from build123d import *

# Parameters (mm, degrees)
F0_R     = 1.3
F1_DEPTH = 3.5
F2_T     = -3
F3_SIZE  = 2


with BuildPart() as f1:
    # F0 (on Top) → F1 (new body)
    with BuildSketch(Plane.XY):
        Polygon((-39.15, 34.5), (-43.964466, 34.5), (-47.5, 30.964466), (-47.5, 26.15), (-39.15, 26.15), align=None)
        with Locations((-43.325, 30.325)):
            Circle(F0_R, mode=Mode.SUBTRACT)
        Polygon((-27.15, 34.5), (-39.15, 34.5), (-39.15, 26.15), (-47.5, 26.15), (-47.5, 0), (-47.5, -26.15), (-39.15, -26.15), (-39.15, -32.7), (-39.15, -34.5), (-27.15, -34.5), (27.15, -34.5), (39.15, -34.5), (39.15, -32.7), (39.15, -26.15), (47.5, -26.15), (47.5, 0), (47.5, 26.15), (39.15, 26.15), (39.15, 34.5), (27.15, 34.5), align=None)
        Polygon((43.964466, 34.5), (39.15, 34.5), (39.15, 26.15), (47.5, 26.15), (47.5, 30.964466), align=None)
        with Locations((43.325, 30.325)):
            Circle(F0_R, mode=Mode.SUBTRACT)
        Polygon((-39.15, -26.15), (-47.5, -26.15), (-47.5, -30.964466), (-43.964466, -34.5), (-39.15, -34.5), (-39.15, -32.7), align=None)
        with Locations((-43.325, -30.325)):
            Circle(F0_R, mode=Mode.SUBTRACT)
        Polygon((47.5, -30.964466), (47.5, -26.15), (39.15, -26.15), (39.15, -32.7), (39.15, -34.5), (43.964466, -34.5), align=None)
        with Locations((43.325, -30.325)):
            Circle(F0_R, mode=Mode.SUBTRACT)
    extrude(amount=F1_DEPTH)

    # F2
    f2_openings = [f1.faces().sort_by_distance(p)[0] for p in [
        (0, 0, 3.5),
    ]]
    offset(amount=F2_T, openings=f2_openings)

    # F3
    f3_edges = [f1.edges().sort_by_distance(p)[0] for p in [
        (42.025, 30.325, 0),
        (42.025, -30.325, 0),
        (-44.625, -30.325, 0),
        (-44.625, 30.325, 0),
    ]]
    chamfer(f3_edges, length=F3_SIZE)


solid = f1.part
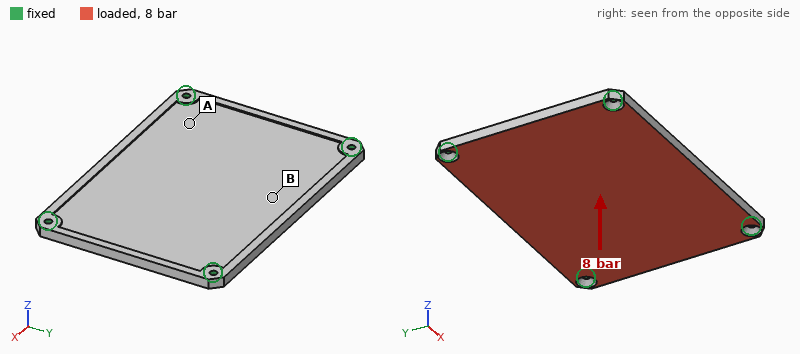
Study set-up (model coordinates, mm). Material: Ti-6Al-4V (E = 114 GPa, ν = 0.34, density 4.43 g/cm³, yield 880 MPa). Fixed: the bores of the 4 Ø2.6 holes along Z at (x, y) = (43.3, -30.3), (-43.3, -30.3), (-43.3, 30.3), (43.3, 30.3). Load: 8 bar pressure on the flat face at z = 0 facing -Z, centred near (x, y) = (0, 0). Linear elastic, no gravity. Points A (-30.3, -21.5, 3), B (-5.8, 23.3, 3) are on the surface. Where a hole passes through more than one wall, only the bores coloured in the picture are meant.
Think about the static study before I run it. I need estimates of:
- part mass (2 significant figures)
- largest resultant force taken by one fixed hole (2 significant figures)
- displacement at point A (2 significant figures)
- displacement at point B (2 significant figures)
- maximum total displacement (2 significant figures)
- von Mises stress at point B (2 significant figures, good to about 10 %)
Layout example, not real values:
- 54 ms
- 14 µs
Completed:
- 88 g
- 3.4 kN
- 0.37 mm
- 0.82 mm
- 0.92 mm
- 180 MPa
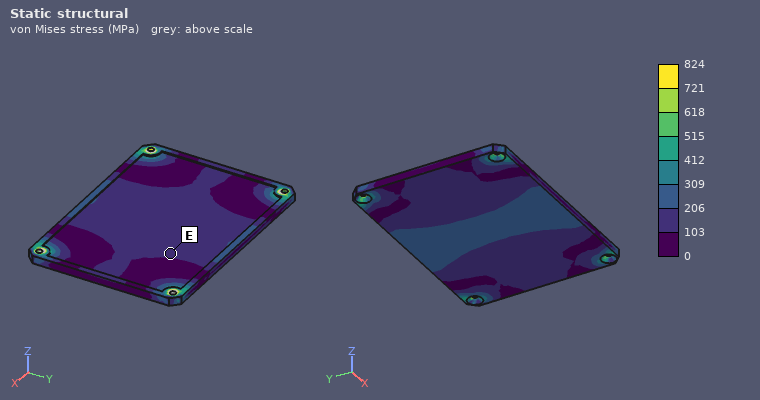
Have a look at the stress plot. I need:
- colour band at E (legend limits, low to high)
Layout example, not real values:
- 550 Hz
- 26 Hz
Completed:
- 103 to 206 MPa
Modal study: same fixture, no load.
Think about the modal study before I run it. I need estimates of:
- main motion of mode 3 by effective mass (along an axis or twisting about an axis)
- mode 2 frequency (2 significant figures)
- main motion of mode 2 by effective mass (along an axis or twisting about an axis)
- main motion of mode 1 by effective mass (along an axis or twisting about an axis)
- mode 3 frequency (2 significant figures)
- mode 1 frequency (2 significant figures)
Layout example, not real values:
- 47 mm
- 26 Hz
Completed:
- twisting about Y
- 2500 Hz
- twisting about X
- along Z
- 3500 Hz
- 1500 Hz
